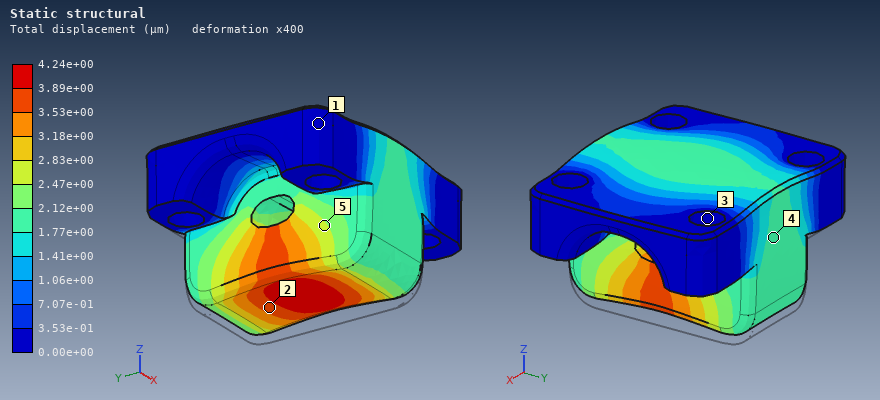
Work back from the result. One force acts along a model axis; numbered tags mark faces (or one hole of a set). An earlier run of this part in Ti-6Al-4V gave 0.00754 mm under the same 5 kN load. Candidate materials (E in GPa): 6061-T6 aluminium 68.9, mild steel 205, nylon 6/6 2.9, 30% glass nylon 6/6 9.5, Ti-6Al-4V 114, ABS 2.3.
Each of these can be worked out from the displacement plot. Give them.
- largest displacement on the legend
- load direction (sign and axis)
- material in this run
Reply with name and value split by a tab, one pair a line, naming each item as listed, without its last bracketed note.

largest displacement on the legend	4.24e+00 µm
load direction	+Z
material in this run	mild steel
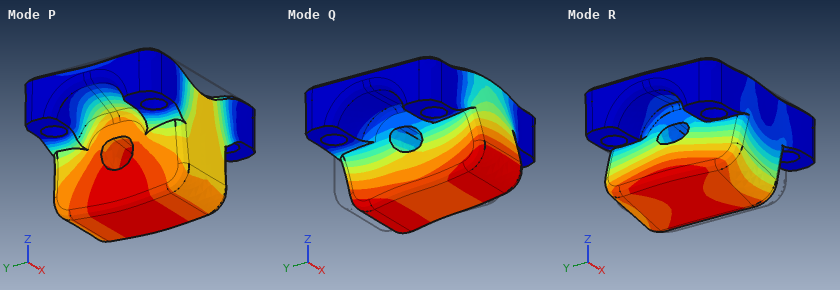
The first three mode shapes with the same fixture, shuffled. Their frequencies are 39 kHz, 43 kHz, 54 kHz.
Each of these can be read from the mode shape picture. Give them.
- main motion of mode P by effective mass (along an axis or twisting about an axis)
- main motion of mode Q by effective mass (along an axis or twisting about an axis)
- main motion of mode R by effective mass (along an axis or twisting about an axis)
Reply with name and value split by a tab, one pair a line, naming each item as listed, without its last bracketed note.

main motion of mode P by effective mass	along Z
main motion of mode Q by effective mass	along Y
main motion of mode R by effective mass	along X
